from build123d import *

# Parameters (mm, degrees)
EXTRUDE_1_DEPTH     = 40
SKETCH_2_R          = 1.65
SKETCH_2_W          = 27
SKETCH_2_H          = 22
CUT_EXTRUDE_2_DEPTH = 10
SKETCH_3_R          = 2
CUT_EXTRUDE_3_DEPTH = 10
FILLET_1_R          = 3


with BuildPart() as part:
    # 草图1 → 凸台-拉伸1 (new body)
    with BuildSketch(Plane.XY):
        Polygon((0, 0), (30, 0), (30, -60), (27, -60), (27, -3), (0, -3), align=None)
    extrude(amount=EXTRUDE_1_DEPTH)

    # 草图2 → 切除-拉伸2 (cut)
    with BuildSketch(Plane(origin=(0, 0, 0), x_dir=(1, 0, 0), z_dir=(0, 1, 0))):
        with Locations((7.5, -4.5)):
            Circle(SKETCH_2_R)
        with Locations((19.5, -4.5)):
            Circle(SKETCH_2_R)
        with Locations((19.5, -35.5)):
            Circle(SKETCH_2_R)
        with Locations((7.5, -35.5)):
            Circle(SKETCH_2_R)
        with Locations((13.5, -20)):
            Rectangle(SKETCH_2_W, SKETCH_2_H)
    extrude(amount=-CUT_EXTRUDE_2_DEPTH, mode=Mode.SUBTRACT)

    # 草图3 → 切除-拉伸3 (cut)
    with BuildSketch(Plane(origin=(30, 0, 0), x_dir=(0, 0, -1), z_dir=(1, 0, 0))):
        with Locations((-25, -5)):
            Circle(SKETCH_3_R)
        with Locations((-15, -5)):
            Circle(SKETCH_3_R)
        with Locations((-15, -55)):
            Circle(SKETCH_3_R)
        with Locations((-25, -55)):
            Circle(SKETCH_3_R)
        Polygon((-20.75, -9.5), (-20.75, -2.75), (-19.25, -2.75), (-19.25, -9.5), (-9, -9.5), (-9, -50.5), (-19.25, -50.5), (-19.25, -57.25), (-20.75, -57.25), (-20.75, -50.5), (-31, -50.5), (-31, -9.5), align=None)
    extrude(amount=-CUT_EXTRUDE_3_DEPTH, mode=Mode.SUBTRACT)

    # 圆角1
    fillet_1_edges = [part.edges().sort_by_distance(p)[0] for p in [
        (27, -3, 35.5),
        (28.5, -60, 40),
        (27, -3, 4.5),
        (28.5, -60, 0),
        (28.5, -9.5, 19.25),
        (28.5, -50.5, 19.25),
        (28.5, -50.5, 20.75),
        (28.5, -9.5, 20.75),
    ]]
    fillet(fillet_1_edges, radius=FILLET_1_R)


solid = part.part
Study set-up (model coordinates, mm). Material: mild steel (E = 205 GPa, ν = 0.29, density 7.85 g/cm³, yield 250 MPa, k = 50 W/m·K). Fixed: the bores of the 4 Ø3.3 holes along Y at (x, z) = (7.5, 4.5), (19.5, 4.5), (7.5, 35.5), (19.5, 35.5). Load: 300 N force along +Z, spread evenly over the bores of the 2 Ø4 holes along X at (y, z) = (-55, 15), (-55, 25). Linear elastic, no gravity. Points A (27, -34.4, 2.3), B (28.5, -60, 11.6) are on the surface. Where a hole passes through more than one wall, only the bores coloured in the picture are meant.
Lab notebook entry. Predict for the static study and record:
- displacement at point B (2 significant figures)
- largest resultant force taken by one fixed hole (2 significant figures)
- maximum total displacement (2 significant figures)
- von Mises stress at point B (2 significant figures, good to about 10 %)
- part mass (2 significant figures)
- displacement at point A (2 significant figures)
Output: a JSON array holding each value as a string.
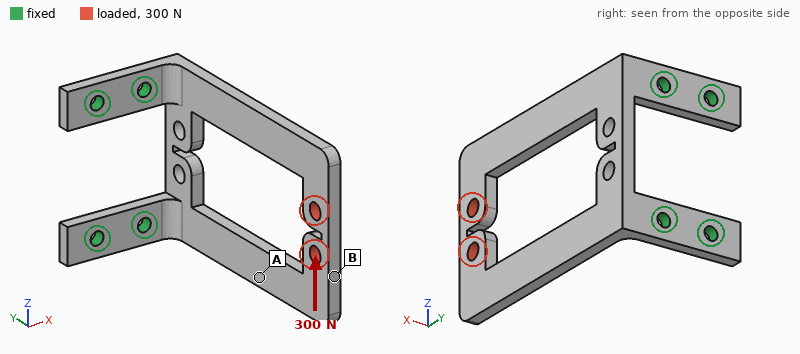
["0.13 mm", "490 N", "0.14 mm", "58 MPa", "44 g", "0.086 mm"]
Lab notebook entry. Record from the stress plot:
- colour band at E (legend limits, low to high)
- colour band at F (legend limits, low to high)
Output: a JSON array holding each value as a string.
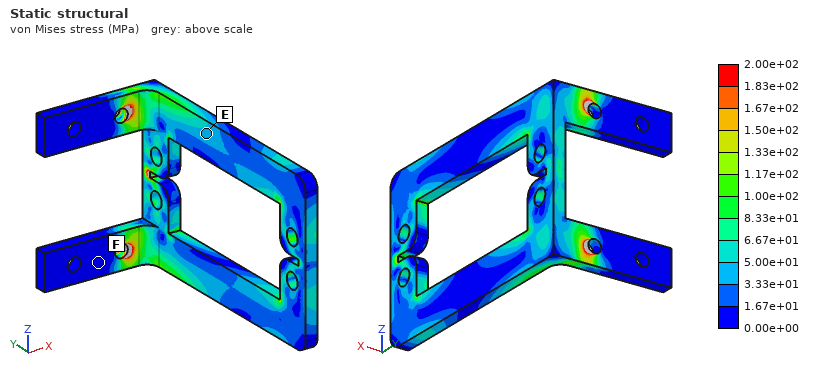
["3.33e+01 to 5.00e+01 MPa", "0.00e+00 to 1.67e+01 MPa"]
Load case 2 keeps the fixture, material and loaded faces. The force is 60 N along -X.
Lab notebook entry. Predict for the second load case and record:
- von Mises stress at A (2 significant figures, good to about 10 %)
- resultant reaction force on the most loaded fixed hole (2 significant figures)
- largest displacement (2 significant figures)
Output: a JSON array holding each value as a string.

["46 MPa", "30 N", "0.51 mm"]
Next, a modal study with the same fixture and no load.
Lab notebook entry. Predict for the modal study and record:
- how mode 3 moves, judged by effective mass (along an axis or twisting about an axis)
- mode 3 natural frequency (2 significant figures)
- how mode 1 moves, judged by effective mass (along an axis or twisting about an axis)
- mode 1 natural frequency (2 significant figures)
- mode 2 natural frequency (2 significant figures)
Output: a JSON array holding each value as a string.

["along Z", "2200 Hz", "along X", "530 Hz", "1600 Hz"]
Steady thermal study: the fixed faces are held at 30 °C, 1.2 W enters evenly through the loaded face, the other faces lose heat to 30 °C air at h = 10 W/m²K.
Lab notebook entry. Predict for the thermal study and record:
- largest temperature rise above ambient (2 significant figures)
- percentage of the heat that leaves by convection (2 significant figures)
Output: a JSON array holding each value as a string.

["23 K", "35 %"]
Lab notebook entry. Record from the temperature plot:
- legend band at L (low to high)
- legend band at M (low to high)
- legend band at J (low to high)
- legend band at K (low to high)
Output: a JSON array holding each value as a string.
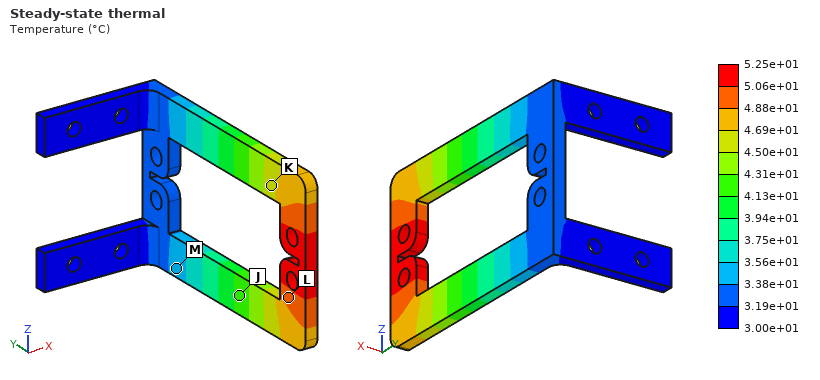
["4.88e+01 to 5.06e+01 °C", "3.38e+01 to 3.56e+01 °C", "4.13e+01 to 4.31e+01 °C", "4.50e+01 to 4.69e+01 °C"]
